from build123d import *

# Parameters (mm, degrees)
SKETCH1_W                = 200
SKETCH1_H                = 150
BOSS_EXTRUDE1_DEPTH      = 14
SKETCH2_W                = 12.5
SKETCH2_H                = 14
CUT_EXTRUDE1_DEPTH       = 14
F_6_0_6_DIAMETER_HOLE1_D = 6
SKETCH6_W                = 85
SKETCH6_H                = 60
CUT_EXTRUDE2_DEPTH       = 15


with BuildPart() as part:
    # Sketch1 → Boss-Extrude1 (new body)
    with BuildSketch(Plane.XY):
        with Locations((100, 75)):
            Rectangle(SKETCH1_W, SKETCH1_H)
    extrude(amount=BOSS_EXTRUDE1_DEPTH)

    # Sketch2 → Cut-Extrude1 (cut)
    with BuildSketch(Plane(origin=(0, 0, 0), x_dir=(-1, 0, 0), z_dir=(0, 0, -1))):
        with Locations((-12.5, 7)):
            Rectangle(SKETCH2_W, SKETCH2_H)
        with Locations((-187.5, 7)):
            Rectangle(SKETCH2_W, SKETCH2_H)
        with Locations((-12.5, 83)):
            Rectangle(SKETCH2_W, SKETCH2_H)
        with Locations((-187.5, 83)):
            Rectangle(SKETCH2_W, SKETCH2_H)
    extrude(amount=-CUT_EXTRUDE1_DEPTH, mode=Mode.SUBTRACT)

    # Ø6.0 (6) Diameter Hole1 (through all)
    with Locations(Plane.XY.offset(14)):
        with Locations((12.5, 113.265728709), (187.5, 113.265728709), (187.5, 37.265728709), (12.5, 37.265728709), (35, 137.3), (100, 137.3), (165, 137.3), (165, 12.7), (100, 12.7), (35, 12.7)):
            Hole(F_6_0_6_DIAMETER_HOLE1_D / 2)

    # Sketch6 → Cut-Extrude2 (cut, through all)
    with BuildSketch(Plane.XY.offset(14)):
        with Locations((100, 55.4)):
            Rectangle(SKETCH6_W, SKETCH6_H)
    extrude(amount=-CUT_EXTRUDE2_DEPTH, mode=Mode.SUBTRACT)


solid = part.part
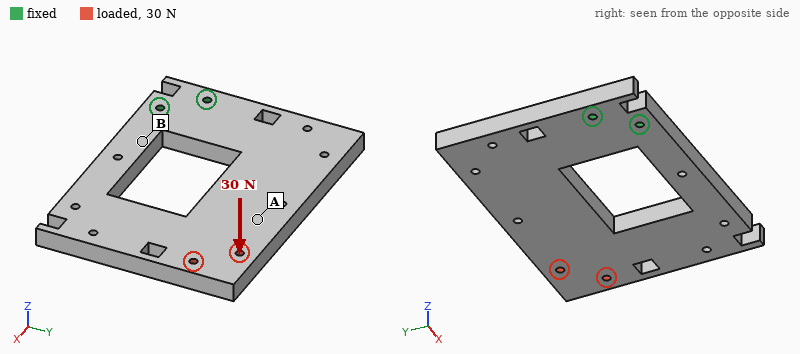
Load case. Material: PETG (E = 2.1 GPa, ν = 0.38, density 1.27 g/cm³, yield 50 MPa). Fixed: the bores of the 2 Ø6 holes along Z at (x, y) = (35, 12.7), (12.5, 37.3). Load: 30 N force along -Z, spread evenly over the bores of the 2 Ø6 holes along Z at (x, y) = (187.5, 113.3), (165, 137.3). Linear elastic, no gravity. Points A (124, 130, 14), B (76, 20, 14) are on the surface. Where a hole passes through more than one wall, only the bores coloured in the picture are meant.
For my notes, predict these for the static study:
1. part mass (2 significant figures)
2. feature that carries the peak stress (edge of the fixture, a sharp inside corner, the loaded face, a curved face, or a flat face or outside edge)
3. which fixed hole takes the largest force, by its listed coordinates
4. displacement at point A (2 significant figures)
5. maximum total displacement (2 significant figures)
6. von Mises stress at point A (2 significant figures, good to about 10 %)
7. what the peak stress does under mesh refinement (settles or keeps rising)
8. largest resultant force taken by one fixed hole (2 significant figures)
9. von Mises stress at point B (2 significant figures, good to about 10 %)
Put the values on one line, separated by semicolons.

430 g; edge of the fixture; (35, 12.7); 1.3 mm; 2.3 mm; 0.51 MPa; keeps rising; 28 N; 1.7 MPa
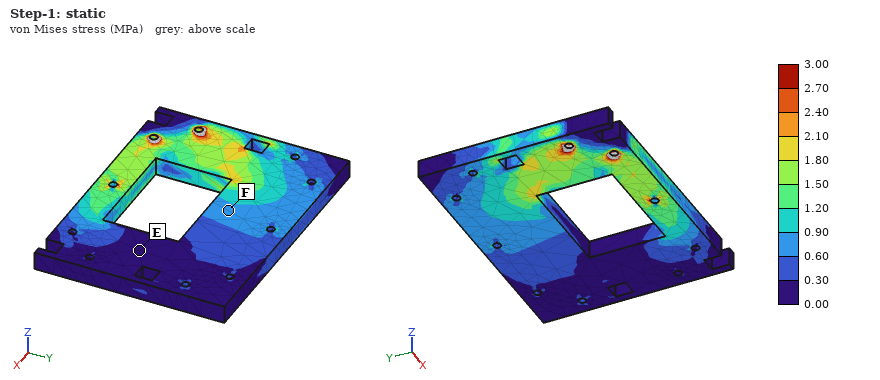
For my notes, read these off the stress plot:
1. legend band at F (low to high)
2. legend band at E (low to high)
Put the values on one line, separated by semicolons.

0.60 to 0.90 MPa; 0.00 to 0.30 MPa
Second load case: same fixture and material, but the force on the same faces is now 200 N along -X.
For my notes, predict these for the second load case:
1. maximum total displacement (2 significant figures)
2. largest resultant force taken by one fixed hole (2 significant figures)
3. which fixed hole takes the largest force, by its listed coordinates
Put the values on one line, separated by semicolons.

0.43 mm; 610 N; (12.5, 37.3)
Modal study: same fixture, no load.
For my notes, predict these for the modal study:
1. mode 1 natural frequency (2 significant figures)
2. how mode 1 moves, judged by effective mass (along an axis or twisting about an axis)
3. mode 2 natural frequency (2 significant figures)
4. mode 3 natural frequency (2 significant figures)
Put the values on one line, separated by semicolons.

58 Hz; along Z; 140 Hz; 190 Hz
